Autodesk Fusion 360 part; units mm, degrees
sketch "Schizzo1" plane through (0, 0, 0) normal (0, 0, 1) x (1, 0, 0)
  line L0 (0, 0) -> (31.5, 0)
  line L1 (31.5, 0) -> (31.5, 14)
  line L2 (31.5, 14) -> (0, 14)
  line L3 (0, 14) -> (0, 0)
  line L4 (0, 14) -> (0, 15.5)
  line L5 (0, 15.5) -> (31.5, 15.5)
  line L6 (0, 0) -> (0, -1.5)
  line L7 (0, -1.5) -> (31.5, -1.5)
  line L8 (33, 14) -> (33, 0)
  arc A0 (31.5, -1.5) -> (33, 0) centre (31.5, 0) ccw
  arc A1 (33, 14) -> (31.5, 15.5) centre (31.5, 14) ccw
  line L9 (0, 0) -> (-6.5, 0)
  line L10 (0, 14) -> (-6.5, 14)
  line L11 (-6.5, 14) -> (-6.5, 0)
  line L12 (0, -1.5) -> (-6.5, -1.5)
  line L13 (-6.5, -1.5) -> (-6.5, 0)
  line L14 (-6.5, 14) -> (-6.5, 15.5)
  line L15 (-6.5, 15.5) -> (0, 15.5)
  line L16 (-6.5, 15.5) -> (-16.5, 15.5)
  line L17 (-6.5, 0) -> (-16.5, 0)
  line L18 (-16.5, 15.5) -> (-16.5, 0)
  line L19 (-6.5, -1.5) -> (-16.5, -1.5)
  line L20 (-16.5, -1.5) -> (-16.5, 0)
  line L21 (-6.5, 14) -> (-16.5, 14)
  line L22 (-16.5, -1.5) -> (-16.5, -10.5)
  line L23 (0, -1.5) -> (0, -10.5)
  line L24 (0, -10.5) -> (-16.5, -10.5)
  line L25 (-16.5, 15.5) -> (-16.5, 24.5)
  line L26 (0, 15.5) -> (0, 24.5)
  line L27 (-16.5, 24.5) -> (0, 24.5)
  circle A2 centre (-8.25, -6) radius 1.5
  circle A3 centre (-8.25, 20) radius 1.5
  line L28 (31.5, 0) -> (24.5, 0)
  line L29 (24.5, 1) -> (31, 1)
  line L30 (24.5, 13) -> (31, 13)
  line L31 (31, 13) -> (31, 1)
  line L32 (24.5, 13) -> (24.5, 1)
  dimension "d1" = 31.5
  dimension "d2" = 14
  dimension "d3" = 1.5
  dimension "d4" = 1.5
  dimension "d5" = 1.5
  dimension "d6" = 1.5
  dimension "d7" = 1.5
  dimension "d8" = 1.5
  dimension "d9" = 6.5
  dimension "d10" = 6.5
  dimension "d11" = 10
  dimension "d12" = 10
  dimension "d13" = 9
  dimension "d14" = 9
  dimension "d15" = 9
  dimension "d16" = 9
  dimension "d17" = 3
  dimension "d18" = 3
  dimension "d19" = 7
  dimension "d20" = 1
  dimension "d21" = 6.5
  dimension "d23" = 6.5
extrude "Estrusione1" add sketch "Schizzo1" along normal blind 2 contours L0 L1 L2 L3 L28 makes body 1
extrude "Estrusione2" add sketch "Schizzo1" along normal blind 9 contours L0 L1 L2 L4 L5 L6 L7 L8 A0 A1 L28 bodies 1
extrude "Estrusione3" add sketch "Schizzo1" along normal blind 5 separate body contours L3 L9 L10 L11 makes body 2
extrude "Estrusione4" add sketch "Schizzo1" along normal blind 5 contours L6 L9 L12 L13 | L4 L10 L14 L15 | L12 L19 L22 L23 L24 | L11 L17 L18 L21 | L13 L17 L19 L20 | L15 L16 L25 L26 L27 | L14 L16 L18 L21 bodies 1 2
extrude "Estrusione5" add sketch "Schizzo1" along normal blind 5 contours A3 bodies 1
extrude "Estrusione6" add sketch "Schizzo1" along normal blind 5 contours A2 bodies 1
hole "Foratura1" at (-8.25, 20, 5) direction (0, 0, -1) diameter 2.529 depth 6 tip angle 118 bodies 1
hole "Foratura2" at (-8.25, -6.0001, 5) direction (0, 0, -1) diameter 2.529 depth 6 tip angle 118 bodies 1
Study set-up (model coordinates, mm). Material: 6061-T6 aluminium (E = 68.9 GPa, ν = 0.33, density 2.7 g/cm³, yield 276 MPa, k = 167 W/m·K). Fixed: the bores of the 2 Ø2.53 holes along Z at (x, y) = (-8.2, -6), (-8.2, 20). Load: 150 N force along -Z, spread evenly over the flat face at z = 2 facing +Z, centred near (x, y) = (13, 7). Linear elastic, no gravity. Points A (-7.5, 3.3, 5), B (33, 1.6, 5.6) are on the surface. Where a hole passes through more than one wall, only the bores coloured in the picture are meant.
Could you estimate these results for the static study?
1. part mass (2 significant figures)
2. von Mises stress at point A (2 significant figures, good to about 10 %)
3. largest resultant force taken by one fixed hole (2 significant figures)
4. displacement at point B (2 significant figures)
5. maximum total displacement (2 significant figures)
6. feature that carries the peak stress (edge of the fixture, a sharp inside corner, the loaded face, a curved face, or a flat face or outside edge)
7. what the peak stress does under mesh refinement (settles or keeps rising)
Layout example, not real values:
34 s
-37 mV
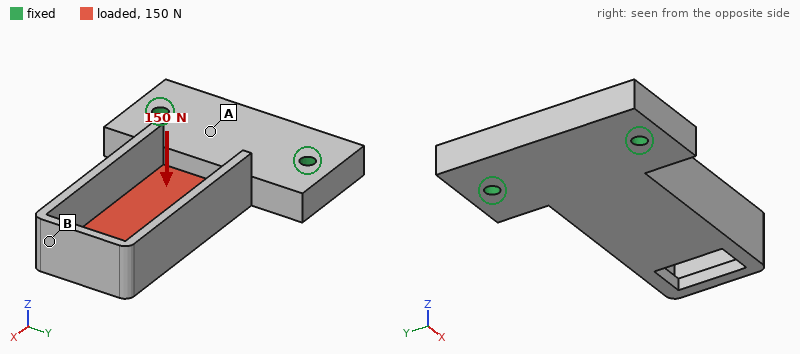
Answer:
13 g
12 MPa
75 N
0.13 mm
0.13 mm
a sharp inside corner
keeps rising
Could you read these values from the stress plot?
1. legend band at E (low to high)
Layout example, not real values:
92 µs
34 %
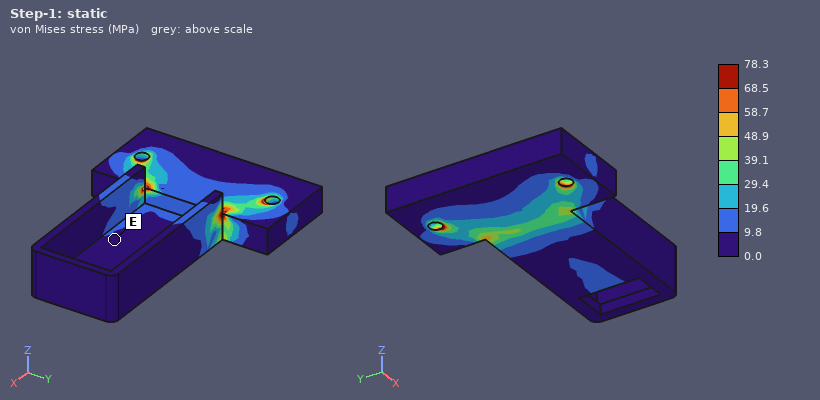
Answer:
0.0 to 9.8 MPa
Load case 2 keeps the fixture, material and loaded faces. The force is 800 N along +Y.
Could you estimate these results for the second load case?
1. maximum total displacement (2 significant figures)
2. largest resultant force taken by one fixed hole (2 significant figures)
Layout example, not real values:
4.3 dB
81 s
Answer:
0.15 mm
770 N
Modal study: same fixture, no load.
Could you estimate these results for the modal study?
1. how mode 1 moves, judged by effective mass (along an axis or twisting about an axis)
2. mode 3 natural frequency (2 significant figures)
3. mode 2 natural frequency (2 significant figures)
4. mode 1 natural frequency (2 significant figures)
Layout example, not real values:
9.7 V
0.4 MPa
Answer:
along Z
8800 Hz
4100 Hz
2600 Hz
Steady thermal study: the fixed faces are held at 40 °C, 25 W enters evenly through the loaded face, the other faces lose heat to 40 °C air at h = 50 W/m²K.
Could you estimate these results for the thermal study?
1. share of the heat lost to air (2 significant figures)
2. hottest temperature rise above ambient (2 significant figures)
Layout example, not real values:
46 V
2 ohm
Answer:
16 %
46 K
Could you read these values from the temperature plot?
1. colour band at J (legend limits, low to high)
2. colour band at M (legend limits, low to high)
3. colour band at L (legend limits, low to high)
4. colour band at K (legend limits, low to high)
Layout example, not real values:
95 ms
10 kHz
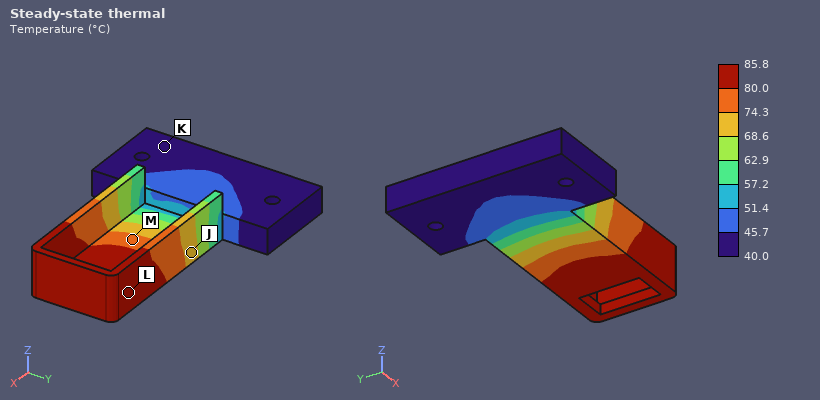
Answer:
68.6 to 74.3 °C
74.3 to 80.0 °C
80.0 to 85.8 °C
40.0 to 45.7 °C
